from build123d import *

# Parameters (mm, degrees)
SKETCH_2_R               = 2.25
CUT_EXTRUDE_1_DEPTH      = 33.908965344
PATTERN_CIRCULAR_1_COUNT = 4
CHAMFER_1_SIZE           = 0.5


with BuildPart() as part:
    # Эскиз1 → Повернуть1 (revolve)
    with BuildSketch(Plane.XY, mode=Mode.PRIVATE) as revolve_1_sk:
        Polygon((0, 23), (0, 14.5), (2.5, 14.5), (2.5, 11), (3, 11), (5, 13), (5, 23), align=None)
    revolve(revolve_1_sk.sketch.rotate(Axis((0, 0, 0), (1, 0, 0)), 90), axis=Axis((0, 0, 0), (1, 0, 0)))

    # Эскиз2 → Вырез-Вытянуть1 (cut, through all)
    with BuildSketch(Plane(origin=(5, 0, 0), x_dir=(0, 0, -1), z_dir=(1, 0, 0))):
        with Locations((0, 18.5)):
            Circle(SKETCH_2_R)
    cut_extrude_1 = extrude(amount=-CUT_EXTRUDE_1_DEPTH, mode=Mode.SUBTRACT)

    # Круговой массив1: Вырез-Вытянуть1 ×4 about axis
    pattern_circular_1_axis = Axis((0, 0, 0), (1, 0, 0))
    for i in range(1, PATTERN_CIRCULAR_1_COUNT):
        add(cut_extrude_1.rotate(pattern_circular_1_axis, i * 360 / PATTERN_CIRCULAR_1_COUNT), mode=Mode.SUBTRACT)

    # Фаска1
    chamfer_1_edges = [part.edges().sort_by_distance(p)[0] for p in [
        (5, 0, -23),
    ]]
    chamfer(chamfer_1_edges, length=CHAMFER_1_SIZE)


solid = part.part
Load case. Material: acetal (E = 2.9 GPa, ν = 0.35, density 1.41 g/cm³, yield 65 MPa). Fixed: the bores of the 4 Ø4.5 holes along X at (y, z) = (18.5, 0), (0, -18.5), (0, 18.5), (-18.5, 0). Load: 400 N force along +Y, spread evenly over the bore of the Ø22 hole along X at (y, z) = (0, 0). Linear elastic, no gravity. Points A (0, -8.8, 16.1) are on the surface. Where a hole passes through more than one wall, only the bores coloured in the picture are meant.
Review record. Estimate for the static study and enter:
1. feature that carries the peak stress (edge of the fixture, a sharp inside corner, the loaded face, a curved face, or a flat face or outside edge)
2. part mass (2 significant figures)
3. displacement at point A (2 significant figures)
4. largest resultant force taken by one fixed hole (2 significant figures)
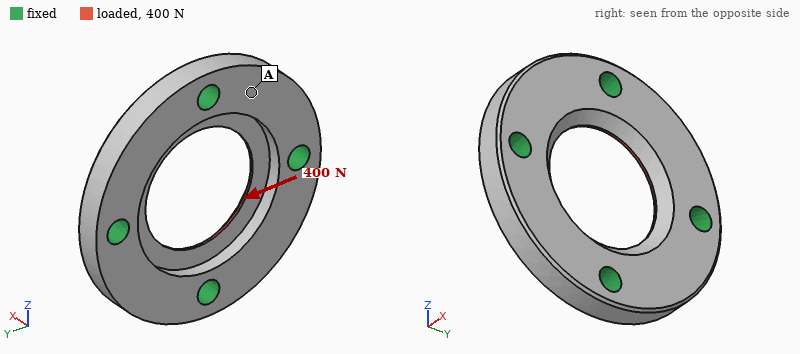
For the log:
the loaded face
7.4 g
4.6 µm
110 N
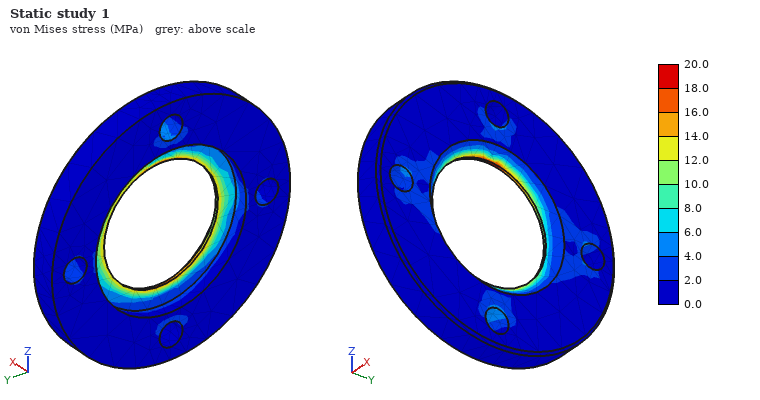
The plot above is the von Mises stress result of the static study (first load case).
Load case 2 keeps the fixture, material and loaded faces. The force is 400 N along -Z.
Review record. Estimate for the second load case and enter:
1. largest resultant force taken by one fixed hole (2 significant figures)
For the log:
110 N
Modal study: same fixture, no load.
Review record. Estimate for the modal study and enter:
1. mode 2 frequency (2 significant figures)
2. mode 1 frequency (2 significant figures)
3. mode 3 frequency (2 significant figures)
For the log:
7800 Hz
7700 Hz
7800 Hz
